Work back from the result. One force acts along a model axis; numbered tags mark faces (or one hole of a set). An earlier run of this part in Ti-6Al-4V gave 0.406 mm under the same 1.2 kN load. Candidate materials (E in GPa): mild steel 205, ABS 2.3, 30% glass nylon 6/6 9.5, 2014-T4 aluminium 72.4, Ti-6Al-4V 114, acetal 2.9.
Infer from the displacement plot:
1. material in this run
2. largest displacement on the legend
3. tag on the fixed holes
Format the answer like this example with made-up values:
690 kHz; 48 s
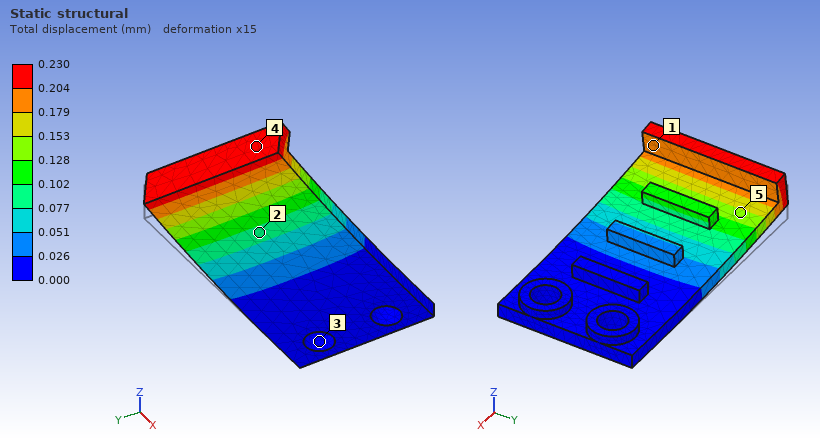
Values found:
mild steel; 0.230 mm; 3
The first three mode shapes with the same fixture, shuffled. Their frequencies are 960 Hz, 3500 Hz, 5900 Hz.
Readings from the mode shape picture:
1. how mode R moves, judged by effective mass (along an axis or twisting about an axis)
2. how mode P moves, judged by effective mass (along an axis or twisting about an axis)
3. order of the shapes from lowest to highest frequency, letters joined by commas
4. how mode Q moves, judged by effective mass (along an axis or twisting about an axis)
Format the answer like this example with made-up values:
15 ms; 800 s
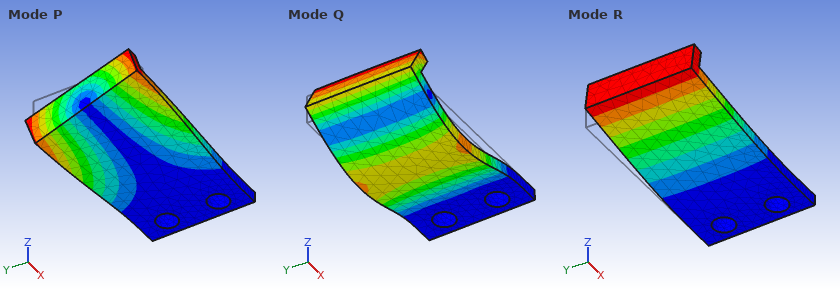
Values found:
along Z; twisting about X; R, P, Q; along Z
